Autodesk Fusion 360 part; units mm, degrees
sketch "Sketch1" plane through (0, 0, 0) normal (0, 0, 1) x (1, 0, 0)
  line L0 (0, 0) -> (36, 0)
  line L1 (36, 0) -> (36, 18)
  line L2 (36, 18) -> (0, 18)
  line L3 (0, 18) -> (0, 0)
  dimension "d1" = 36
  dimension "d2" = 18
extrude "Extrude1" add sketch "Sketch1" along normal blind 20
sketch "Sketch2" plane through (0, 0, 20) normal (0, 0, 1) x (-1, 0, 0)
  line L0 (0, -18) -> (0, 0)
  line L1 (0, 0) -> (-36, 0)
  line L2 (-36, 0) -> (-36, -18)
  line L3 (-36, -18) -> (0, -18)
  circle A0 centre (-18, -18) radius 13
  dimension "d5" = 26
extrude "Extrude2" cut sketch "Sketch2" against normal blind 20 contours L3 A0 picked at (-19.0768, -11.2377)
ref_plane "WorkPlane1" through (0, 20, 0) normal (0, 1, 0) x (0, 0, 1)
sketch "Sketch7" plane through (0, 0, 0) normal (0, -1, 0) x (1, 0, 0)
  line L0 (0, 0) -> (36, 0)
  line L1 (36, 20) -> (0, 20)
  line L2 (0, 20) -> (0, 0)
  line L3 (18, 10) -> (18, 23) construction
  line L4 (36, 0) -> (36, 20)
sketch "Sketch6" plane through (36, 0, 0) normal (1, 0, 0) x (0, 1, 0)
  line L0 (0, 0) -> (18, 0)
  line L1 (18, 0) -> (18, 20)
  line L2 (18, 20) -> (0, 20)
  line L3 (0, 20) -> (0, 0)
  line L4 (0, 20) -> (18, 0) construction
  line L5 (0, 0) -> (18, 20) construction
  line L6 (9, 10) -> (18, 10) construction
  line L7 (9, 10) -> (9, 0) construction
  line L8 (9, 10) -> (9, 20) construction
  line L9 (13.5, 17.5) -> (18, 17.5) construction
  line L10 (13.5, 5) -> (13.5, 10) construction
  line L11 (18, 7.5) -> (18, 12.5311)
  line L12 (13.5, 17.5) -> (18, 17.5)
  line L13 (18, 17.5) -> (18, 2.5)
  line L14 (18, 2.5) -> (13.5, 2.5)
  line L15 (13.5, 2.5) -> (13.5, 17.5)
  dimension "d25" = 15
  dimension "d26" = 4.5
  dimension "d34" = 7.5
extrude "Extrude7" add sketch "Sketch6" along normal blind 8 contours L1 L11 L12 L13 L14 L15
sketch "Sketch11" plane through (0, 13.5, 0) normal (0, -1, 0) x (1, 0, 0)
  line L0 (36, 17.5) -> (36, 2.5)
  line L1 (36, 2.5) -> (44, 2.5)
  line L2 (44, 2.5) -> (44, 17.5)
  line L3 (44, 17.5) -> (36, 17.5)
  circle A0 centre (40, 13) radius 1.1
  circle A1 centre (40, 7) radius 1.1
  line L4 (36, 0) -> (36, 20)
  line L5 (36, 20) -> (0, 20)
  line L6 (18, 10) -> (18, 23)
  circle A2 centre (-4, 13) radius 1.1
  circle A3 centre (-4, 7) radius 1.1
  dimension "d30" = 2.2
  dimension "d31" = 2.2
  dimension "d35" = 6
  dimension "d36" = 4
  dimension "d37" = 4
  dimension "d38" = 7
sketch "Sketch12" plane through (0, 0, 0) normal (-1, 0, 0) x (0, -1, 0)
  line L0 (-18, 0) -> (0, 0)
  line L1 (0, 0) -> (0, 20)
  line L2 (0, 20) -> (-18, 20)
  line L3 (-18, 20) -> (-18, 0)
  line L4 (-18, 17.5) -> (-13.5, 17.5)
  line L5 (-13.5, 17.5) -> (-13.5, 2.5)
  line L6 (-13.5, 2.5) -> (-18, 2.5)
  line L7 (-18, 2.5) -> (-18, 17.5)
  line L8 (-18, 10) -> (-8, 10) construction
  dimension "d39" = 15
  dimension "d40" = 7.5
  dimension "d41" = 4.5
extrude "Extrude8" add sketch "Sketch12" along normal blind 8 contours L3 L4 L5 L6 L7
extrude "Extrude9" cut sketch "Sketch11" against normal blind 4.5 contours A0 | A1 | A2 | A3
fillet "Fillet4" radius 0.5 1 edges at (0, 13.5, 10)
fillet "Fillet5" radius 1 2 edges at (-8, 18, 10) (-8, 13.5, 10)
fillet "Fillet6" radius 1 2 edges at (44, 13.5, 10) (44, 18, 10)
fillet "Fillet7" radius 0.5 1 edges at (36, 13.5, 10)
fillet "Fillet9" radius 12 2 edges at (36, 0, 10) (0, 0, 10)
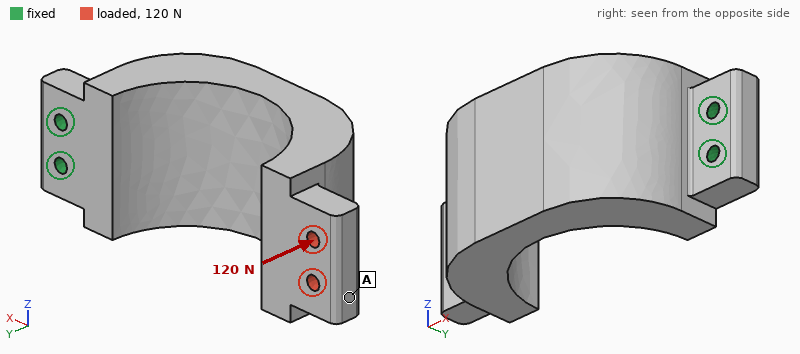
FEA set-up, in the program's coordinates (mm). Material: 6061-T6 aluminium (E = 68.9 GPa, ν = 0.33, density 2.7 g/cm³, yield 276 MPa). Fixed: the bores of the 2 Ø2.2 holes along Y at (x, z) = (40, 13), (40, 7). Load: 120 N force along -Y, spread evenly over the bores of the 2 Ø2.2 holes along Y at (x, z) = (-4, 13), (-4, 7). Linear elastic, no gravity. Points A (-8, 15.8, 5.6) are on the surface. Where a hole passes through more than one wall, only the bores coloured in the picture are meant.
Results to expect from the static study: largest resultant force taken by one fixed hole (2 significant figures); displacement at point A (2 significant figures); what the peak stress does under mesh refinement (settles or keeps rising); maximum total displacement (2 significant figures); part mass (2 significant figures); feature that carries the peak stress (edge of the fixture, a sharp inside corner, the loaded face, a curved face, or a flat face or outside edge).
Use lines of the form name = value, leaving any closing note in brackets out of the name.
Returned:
largest resultant force taken by one fixed hole = 74 N
displacement at point A = 0.29 mm
what the peak stress does under mesh refinement = keeps rising
maximum total displacement = 0.29 mm
part mass = 20 g
feature that carries the peak stress = edge of the fixture
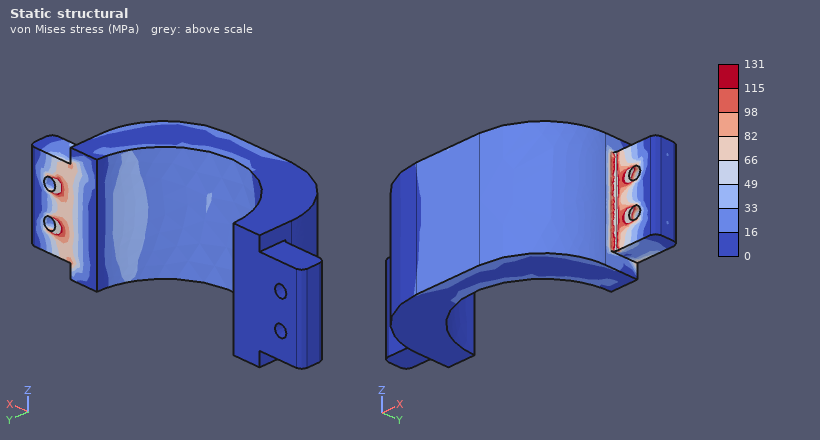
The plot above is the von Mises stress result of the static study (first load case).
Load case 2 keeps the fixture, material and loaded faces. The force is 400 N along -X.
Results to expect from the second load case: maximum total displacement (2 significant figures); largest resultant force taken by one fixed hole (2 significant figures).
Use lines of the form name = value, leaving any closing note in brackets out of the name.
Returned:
maximum total displacement = 0.18 mm
largest resultant force taken by one fixed hole = 200 N
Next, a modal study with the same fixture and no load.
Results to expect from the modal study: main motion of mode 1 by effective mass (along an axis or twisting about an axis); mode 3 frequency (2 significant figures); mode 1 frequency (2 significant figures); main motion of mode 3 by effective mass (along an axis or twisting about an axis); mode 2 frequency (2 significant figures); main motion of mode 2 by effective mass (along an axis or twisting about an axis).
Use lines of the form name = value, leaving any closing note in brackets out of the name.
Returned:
main motion of mode 1 by effective mass = along Y
mode 3 frequency = 5100 Hz
mode 1 frequency = 1400 Hz
main motion of mode 3 by effective mass = along X
mode 2 frequency = 2600 Hz
main motion of mode 2 by effective mass = along Z
